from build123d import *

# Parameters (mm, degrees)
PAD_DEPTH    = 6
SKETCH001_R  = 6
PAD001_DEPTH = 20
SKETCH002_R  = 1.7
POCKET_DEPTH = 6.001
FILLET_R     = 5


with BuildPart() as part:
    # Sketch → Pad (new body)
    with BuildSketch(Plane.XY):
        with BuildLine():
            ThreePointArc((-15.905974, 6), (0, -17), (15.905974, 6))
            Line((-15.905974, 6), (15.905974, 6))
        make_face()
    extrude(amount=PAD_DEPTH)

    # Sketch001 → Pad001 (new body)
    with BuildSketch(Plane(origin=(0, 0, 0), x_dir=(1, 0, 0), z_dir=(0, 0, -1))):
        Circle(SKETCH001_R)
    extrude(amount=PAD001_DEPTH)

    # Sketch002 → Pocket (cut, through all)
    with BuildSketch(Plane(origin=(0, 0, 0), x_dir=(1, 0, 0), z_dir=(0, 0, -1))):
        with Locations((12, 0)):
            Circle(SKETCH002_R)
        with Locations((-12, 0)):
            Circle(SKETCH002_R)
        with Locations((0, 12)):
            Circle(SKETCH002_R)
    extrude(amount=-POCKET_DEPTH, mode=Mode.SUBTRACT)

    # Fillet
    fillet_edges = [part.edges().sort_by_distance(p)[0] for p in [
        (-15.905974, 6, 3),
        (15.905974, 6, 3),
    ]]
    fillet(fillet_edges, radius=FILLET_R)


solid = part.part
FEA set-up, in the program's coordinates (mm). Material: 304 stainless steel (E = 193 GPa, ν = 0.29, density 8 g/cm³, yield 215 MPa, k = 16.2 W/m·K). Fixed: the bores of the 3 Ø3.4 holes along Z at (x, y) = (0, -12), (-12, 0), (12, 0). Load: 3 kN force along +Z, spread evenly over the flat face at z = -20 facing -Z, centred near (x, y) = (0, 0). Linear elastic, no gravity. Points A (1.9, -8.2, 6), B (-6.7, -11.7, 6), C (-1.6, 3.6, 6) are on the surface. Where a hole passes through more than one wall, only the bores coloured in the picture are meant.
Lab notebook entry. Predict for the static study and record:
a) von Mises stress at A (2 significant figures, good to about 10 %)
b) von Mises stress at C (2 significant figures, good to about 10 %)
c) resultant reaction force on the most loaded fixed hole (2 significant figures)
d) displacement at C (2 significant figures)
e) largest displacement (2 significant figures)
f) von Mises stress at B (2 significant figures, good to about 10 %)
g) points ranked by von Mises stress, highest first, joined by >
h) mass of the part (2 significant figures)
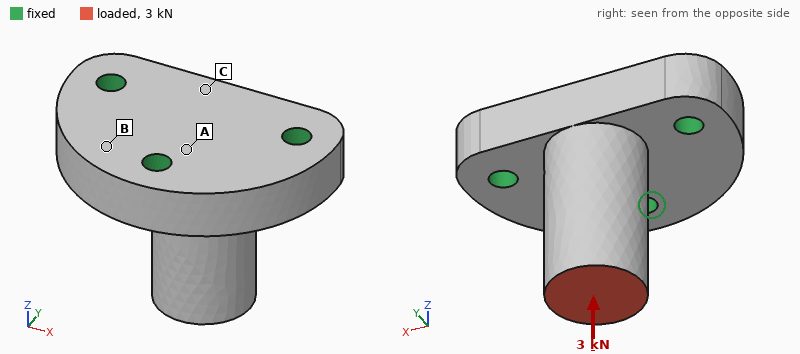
23 MPa
44 MPa
1.2 kN
4.9 µm
11 µm
11 MPa
C > A > B
48 g
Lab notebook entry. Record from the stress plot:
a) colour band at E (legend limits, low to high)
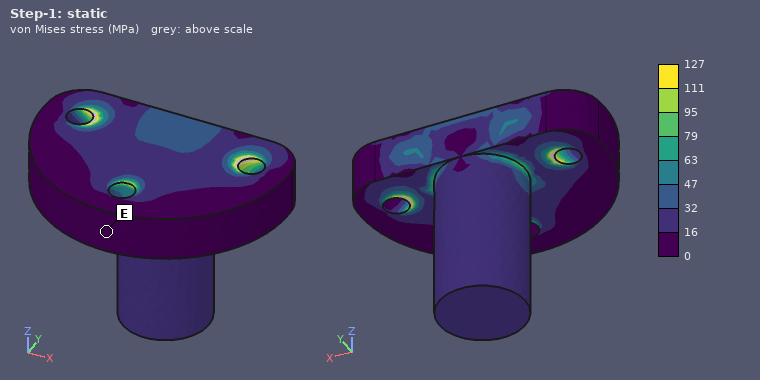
0 to 16 MPa
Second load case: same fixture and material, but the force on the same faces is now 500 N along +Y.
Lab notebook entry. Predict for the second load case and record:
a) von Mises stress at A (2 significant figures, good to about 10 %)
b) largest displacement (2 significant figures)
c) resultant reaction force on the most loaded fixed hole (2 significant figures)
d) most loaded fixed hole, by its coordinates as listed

12 MPa
20 µm
750 N
(0, -12)
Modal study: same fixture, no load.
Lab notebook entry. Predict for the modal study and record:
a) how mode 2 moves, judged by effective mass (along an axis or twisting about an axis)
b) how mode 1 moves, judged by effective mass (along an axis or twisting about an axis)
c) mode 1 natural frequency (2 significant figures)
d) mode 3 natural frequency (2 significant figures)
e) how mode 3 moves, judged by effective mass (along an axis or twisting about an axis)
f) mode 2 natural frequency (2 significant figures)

along X
along Y
10 kHz
28 kHz
along Z
13 kHz
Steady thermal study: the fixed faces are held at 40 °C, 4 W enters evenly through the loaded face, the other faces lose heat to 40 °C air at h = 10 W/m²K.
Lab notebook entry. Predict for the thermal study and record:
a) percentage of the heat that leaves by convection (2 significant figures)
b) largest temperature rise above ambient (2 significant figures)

7.3 %
54 K
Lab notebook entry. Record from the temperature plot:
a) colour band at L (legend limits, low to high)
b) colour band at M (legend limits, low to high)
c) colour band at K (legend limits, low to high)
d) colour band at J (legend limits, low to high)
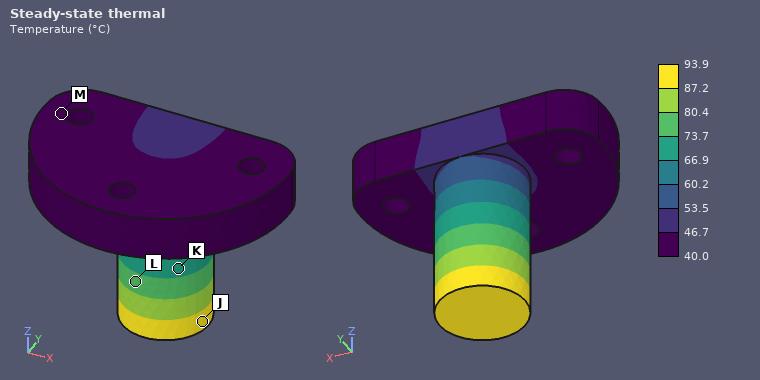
73.7 to 80.4 °C
40.0 to 46.7 °C
66.9 to 73.7 °C
87.2 to 93.9 °C
